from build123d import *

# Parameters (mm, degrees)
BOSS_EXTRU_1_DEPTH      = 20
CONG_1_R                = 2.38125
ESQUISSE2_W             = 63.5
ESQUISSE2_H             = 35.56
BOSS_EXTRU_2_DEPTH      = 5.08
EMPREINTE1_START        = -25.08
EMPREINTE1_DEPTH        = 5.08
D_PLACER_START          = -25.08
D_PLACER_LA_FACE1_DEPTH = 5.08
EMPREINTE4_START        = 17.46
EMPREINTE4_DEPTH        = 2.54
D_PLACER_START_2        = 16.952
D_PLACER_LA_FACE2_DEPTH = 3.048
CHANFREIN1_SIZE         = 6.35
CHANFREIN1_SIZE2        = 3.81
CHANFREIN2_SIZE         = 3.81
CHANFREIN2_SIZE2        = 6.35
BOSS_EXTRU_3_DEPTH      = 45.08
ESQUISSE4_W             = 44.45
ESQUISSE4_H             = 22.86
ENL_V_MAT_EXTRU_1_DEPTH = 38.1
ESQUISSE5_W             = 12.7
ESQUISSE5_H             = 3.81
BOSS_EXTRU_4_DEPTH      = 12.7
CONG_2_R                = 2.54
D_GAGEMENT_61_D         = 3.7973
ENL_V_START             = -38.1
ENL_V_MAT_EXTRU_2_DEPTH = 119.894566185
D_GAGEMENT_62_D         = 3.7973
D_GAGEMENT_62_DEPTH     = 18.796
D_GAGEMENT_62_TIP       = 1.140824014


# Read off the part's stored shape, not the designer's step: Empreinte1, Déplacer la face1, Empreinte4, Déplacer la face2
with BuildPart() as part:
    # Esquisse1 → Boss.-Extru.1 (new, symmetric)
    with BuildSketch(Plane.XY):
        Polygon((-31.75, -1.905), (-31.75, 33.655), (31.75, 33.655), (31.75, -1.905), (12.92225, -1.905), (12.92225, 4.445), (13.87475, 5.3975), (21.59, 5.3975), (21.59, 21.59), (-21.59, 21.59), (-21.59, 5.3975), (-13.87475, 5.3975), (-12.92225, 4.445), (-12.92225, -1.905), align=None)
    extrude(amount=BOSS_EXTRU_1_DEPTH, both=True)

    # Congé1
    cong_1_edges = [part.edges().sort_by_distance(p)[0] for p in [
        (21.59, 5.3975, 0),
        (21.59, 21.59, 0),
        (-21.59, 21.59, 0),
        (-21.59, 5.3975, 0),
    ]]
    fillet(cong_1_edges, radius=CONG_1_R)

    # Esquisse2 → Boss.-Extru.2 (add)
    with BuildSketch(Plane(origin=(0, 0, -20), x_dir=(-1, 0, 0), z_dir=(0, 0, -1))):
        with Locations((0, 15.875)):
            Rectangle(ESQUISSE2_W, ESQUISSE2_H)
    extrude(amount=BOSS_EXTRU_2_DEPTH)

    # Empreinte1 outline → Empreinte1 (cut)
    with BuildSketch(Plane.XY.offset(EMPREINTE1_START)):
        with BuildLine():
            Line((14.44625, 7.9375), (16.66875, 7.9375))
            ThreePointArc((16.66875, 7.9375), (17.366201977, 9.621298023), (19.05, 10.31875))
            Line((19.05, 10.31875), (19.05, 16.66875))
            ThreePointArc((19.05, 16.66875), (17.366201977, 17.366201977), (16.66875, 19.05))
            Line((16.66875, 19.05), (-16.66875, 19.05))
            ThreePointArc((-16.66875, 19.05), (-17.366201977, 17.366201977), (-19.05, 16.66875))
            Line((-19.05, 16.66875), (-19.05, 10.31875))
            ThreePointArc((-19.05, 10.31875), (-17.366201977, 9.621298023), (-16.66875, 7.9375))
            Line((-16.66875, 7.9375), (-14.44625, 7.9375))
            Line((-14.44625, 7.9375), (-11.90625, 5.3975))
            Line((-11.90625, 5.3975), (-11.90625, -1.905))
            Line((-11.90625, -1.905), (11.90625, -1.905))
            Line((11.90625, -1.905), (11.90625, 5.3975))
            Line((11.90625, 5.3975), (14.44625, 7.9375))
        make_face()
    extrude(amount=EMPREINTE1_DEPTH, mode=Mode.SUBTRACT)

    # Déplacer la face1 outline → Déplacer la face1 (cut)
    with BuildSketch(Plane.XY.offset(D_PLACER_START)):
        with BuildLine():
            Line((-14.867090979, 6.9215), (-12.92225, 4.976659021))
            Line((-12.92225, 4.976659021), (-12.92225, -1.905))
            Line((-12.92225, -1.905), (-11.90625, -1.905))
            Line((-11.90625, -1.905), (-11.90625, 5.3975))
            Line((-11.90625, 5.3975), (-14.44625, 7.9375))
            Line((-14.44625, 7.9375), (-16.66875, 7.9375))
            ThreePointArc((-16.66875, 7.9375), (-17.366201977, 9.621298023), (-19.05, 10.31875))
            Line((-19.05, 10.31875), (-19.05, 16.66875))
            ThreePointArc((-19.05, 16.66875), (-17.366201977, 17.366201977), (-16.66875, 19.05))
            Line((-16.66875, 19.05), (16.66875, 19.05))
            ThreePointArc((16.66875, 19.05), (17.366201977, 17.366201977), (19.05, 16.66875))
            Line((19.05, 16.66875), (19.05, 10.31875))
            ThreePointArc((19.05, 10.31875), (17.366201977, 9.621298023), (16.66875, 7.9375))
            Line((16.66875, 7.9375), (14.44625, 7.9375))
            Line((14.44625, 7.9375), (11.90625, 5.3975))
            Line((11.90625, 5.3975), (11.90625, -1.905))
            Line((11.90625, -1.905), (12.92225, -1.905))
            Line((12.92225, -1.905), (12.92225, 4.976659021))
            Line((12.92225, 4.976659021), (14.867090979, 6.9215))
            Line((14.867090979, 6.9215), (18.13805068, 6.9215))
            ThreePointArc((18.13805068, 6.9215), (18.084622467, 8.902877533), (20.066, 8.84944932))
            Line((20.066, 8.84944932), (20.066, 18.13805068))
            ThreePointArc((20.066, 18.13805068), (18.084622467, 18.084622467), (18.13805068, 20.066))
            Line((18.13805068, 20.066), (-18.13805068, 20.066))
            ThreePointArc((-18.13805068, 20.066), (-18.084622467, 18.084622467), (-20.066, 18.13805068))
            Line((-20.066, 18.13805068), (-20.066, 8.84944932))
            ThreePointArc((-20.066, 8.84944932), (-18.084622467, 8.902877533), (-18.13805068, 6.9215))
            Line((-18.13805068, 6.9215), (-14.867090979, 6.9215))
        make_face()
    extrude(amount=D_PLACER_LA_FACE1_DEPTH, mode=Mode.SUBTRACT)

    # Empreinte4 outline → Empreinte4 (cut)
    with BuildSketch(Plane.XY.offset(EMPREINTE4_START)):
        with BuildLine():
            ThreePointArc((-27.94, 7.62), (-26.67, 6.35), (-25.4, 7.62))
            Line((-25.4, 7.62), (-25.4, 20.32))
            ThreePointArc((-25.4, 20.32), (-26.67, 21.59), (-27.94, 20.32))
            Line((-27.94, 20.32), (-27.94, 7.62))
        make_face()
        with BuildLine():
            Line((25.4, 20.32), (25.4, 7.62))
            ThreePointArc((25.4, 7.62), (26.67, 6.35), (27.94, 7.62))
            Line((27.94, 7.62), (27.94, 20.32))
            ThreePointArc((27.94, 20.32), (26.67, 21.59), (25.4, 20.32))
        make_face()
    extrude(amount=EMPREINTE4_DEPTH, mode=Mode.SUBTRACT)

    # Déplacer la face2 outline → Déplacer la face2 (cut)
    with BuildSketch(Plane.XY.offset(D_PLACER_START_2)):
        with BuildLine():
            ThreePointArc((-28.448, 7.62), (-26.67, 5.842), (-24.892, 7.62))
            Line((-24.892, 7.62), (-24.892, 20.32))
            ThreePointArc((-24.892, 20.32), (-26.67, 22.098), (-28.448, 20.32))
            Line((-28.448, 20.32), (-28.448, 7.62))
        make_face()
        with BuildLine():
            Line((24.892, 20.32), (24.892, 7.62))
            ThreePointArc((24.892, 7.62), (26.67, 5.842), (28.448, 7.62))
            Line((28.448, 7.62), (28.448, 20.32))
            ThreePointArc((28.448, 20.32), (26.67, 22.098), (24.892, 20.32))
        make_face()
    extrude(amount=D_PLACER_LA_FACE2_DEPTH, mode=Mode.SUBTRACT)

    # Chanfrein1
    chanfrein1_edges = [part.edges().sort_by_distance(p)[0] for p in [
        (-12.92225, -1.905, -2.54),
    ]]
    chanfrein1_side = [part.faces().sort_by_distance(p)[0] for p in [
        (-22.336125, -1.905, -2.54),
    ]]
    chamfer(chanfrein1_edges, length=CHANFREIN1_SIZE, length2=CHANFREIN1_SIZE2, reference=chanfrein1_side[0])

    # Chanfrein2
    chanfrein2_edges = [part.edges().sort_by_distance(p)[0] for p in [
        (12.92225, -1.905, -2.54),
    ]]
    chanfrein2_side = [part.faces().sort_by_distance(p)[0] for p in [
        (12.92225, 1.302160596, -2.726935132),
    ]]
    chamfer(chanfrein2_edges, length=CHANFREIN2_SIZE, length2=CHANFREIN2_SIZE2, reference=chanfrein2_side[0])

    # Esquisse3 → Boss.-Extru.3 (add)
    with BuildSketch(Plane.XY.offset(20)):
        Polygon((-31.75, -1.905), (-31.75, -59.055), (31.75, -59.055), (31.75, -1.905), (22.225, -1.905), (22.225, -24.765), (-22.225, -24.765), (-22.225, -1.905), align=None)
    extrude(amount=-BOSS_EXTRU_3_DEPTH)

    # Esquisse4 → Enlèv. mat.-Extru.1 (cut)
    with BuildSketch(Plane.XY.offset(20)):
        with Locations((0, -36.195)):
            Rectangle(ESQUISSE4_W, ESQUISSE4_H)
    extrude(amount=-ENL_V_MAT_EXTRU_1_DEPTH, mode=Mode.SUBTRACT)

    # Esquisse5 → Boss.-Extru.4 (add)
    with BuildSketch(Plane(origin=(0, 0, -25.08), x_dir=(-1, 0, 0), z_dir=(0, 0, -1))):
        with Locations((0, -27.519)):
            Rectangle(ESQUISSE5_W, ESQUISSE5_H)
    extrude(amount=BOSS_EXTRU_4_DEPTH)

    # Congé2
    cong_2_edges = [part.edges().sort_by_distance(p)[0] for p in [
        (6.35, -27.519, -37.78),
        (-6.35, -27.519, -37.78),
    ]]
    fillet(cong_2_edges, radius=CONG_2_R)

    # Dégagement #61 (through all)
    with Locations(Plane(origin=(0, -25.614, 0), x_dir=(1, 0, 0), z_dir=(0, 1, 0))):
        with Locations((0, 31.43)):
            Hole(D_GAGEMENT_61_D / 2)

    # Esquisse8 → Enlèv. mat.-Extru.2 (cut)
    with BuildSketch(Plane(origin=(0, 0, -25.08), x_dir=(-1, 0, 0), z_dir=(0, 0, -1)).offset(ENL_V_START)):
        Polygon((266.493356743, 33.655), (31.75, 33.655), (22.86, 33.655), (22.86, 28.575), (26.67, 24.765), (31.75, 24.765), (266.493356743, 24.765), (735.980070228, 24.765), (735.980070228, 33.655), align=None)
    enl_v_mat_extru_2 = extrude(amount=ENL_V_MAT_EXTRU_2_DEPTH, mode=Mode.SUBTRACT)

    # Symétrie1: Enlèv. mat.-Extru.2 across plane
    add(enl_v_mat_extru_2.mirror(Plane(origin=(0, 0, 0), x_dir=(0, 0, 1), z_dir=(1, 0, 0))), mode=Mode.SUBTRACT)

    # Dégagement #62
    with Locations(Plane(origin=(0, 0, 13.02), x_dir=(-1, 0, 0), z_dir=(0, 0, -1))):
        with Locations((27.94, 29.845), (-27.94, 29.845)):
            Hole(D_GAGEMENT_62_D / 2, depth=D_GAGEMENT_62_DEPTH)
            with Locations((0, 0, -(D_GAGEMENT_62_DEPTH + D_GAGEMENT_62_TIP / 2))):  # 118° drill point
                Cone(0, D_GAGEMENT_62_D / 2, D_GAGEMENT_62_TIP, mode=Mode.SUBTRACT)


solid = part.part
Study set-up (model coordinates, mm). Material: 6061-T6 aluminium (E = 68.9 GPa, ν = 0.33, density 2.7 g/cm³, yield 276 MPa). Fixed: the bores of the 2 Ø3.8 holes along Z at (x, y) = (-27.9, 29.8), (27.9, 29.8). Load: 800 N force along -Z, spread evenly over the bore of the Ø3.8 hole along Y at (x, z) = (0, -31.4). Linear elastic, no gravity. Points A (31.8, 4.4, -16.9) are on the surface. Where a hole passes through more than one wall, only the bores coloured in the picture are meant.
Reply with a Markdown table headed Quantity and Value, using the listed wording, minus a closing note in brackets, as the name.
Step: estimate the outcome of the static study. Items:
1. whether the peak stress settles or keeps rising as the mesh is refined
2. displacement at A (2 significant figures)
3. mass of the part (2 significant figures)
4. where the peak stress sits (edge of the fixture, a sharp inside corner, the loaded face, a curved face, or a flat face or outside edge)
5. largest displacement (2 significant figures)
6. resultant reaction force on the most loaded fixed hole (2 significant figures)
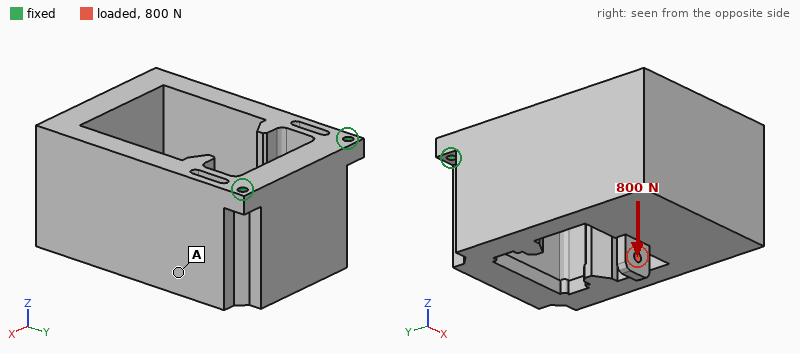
| Quantity | Value |
|---|---|
| whether the peak stress settles or keeps rising as the mesh is refined | keeps rising |
| displacement at A | 0.20 mm |
| mass of the part | 370 g |
| where the peak stress sits | edge of the fixture |
| largest displacement | 0.49 mm |
| resultant reaction force on the most loaded fixed hole | 480 N |
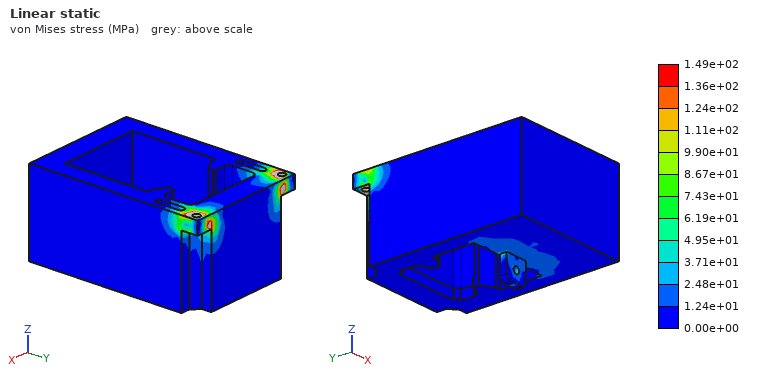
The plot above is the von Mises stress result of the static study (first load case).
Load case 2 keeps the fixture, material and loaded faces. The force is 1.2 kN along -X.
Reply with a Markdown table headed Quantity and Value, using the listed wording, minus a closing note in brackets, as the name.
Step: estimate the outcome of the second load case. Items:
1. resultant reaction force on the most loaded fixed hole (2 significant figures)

| Quantity | Value |
|---|---|
| resultant reaction force on the most loaded fixed hole | 1.7 kN |
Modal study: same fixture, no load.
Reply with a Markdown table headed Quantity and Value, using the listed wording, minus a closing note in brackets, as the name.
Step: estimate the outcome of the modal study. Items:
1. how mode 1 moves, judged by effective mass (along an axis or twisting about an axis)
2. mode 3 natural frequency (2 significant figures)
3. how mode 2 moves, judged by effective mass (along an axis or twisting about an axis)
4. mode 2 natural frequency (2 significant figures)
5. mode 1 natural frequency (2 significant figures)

| Quantity | Value |
|---|---|
| how mode 1 moves, judged by effective mass | along Z |
| mode 3 natural frequency | 2700 Hz |
| how mode 2 moves, judged by effective mass | along X |
| mode 2 natural frequency | 1100 Hz |
| mode 1 natural frequency | 420 Hz |
